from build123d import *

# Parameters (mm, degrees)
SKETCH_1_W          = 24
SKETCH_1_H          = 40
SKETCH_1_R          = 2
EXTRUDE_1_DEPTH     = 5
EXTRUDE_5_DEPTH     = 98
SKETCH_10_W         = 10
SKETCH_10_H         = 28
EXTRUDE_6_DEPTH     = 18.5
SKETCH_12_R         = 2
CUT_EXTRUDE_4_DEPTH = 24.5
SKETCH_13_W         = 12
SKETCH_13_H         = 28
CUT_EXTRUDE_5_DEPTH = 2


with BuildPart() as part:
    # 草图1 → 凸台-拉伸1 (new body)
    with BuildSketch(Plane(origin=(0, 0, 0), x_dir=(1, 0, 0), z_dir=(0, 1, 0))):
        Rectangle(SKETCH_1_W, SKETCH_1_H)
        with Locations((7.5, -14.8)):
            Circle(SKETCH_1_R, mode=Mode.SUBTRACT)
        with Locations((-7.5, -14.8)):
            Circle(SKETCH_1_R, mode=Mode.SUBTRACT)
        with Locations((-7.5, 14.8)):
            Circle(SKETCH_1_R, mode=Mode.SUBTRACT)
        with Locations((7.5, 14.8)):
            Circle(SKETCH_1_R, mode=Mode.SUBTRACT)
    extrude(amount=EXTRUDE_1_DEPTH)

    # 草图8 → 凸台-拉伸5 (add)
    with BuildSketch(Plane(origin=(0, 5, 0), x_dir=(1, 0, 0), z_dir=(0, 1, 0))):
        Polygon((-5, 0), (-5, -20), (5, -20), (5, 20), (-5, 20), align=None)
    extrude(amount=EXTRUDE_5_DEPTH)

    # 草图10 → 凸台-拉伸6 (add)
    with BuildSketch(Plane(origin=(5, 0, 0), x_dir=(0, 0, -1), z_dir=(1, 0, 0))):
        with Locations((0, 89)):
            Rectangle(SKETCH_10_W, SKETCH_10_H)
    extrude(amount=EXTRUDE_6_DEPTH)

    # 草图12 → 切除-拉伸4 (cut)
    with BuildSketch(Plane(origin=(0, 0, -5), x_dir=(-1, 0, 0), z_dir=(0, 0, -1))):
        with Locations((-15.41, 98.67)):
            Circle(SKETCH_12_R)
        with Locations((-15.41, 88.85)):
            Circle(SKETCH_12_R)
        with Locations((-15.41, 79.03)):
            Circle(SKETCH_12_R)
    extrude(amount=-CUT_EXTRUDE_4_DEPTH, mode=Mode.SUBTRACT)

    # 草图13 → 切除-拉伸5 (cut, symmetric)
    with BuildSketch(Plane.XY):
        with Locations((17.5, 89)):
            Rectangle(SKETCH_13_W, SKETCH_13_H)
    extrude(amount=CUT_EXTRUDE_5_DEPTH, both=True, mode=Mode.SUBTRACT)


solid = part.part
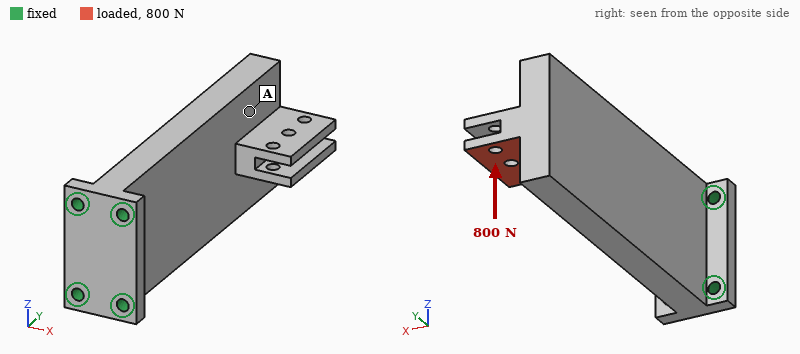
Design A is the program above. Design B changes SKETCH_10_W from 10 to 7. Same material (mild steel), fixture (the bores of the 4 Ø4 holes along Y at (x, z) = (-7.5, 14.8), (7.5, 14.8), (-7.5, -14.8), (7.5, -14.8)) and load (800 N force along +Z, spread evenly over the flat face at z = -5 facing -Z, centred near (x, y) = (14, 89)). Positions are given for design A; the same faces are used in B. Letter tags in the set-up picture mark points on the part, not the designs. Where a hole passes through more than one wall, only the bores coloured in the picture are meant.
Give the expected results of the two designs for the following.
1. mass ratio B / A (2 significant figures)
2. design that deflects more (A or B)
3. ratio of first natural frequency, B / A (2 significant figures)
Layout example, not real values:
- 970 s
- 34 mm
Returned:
- 0.97
- B
- 1.0
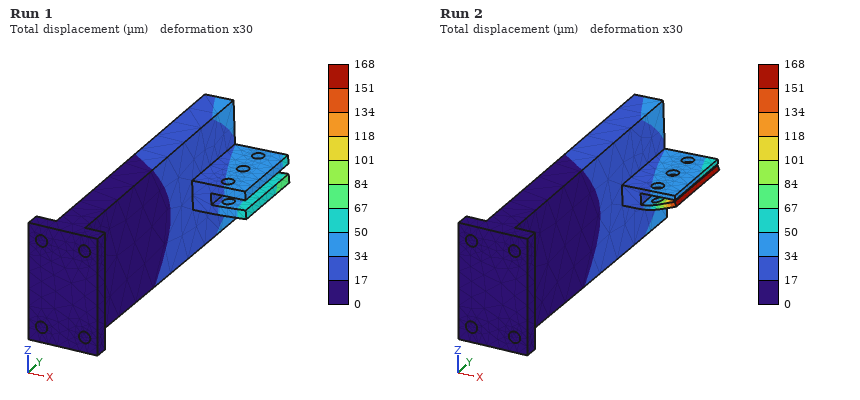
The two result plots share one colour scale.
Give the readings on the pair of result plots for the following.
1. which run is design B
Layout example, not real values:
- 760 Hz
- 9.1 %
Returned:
- Run 2
